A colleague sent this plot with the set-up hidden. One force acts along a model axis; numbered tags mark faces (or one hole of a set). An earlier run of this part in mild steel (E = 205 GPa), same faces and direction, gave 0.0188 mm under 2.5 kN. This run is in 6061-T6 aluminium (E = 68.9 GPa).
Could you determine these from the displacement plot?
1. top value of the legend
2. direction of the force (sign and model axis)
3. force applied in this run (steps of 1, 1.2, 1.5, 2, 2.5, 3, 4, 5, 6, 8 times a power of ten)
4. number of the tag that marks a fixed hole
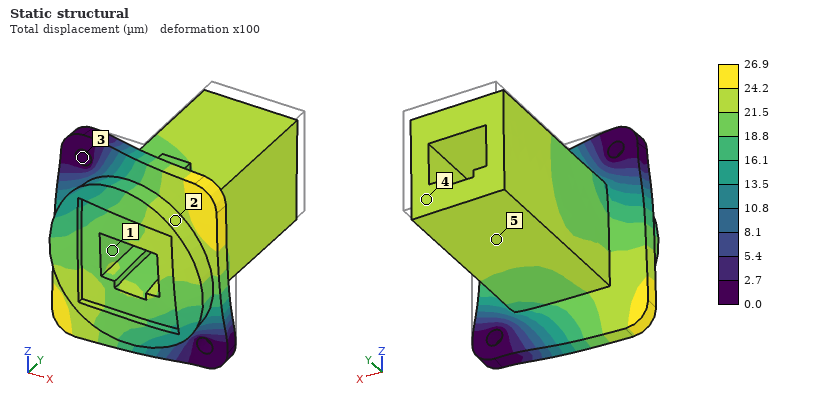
26.9 µm
-Y
1.2 kN
3
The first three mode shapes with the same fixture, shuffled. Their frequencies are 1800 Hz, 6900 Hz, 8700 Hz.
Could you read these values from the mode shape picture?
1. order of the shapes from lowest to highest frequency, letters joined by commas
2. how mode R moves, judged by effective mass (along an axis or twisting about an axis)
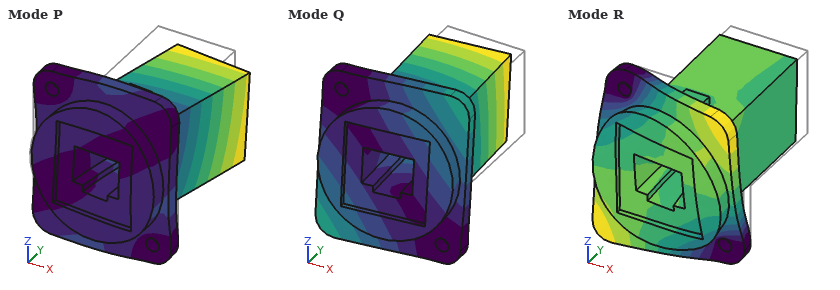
Q, P, R
along Y
